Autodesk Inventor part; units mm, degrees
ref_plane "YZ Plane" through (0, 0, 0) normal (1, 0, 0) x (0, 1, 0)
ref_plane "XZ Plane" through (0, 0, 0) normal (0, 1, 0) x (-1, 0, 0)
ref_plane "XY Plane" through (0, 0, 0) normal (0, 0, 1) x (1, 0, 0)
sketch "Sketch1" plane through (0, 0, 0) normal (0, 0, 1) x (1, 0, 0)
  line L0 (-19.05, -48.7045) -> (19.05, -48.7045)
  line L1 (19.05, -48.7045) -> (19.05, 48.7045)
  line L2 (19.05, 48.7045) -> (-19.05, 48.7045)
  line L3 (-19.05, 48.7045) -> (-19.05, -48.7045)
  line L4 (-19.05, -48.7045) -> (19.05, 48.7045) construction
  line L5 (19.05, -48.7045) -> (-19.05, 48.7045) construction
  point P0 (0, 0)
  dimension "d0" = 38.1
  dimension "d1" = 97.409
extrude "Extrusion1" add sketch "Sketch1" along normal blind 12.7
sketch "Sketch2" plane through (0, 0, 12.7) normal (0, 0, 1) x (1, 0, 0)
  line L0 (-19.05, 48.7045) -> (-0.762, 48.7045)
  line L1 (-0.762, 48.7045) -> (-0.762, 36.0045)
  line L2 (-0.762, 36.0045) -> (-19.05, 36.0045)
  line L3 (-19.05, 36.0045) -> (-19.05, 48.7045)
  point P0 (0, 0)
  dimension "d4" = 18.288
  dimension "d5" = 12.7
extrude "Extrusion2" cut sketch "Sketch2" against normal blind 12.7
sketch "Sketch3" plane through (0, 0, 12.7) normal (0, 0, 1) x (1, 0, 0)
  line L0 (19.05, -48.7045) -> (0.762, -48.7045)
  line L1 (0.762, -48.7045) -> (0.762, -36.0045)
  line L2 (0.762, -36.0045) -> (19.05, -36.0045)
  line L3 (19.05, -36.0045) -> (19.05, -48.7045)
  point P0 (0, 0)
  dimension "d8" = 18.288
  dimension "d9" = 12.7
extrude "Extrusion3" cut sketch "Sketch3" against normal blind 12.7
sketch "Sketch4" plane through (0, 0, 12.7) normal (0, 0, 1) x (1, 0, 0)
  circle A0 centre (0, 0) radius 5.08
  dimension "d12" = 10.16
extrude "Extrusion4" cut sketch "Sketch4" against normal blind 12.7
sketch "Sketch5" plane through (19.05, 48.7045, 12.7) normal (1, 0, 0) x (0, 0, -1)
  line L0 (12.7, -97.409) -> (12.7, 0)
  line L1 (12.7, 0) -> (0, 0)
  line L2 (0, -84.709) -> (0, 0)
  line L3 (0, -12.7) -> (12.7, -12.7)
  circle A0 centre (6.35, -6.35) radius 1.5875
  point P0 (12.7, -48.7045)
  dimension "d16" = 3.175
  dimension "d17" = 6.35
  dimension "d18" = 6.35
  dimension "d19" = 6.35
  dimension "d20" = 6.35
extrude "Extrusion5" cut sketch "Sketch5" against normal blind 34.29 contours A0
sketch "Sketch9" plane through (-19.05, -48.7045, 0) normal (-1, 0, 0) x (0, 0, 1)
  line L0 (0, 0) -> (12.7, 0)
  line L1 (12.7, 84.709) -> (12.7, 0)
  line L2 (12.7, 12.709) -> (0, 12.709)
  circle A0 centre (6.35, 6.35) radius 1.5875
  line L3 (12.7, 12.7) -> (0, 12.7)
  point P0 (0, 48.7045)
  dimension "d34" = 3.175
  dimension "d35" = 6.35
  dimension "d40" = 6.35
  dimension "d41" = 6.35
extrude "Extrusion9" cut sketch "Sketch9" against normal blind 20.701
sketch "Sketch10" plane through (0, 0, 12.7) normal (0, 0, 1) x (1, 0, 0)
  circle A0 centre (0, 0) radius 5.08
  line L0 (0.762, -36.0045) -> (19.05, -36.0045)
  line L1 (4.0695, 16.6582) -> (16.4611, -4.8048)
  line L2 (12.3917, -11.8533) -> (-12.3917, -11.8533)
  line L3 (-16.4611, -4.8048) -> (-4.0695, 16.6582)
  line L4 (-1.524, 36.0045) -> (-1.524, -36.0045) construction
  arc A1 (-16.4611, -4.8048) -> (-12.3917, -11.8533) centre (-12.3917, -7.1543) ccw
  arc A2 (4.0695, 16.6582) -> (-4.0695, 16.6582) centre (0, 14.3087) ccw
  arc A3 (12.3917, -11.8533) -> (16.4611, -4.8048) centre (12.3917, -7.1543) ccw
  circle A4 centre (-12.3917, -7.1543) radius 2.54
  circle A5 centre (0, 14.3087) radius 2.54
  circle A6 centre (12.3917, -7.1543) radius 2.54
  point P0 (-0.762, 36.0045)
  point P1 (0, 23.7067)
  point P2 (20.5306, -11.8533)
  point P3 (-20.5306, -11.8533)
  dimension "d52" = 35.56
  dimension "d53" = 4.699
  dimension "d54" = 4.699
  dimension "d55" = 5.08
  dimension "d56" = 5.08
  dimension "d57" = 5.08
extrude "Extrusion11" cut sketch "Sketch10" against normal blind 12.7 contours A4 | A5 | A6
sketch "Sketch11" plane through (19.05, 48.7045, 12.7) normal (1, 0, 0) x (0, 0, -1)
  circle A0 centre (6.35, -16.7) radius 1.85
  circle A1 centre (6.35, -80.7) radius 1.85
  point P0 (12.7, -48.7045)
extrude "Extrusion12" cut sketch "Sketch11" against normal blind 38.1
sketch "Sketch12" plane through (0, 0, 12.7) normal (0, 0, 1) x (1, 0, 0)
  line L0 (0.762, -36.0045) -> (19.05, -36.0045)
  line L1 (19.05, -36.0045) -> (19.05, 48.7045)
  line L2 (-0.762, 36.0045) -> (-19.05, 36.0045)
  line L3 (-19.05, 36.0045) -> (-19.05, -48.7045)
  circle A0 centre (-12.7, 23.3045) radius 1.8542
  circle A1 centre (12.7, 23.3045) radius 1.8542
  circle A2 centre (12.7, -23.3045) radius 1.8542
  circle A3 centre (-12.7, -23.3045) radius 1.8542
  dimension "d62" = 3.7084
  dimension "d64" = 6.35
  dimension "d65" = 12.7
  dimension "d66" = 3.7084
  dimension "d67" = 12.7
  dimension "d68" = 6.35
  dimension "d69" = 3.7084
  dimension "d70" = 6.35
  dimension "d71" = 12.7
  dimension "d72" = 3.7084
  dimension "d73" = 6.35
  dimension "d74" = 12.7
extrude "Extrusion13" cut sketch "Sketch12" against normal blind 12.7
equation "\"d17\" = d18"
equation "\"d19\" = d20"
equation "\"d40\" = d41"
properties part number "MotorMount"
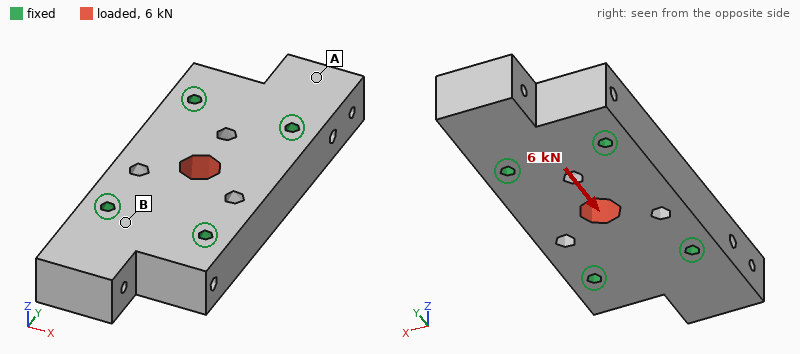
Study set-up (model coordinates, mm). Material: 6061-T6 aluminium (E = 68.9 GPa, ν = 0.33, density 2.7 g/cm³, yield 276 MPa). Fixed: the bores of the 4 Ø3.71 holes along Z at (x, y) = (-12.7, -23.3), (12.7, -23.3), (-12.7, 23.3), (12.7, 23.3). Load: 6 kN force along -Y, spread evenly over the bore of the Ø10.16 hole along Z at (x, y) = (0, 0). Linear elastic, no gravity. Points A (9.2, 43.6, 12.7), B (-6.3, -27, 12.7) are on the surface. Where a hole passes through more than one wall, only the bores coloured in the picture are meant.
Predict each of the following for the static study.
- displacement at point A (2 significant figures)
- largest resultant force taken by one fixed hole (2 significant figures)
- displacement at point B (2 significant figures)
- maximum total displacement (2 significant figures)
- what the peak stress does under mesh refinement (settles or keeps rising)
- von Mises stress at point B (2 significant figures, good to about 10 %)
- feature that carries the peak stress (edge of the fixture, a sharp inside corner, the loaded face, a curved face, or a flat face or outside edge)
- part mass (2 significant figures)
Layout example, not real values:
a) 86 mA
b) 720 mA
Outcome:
a) 0.68 µm
b) 1.6 kN
c) 0.84 µm
d) 4.0 µm
e) keeps rising
f) 4.4 MPa
g) edge of the fixture
h) 100 g
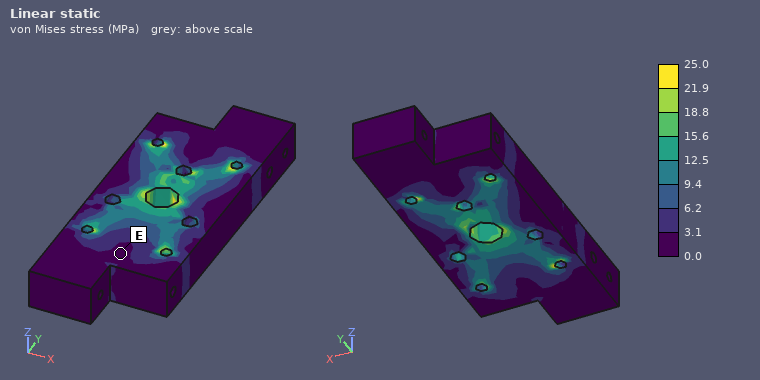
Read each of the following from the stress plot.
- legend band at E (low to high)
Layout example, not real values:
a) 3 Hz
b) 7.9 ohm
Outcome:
a) 0.0 to 3.1 MPa
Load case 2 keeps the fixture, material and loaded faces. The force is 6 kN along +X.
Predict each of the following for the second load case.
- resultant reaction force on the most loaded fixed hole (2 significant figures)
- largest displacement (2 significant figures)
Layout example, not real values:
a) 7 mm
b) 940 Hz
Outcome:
a) 1.9 kN
b) 8.2 µm
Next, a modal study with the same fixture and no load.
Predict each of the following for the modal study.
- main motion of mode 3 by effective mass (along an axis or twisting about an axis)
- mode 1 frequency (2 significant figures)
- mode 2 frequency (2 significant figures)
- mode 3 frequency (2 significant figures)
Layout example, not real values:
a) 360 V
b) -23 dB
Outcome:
a) along Z
b) 13 kHz
c) 14 kHz
d) 20 kHz
